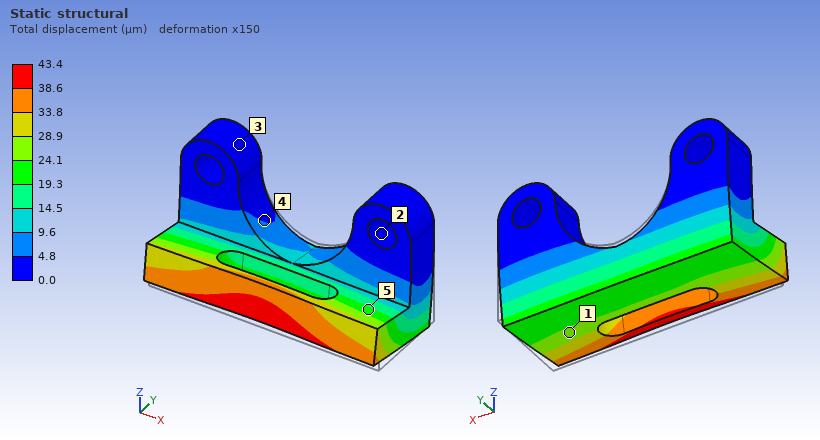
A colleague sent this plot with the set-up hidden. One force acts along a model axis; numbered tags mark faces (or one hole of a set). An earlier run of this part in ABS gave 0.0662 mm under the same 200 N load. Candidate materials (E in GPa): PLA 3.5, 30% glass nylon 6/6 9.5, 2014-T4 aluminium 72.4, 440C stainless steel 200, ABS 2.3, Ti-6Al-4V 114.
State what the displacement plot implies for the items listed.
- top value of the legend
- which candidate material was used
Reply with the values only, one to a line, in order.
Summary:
43.4 µm
PLA
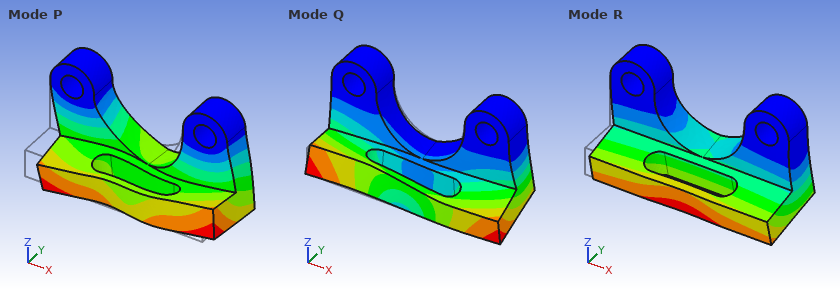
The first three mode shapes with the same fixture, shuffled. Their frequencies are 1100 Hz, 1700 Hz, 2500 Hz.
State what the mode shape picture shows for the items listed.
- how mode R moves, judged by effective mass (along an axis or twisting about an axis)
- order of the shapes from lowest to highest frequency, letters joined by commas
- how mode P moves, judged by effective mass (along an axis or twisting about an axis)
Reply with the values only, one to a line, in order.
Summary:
along Y
R, Q, P
along X
